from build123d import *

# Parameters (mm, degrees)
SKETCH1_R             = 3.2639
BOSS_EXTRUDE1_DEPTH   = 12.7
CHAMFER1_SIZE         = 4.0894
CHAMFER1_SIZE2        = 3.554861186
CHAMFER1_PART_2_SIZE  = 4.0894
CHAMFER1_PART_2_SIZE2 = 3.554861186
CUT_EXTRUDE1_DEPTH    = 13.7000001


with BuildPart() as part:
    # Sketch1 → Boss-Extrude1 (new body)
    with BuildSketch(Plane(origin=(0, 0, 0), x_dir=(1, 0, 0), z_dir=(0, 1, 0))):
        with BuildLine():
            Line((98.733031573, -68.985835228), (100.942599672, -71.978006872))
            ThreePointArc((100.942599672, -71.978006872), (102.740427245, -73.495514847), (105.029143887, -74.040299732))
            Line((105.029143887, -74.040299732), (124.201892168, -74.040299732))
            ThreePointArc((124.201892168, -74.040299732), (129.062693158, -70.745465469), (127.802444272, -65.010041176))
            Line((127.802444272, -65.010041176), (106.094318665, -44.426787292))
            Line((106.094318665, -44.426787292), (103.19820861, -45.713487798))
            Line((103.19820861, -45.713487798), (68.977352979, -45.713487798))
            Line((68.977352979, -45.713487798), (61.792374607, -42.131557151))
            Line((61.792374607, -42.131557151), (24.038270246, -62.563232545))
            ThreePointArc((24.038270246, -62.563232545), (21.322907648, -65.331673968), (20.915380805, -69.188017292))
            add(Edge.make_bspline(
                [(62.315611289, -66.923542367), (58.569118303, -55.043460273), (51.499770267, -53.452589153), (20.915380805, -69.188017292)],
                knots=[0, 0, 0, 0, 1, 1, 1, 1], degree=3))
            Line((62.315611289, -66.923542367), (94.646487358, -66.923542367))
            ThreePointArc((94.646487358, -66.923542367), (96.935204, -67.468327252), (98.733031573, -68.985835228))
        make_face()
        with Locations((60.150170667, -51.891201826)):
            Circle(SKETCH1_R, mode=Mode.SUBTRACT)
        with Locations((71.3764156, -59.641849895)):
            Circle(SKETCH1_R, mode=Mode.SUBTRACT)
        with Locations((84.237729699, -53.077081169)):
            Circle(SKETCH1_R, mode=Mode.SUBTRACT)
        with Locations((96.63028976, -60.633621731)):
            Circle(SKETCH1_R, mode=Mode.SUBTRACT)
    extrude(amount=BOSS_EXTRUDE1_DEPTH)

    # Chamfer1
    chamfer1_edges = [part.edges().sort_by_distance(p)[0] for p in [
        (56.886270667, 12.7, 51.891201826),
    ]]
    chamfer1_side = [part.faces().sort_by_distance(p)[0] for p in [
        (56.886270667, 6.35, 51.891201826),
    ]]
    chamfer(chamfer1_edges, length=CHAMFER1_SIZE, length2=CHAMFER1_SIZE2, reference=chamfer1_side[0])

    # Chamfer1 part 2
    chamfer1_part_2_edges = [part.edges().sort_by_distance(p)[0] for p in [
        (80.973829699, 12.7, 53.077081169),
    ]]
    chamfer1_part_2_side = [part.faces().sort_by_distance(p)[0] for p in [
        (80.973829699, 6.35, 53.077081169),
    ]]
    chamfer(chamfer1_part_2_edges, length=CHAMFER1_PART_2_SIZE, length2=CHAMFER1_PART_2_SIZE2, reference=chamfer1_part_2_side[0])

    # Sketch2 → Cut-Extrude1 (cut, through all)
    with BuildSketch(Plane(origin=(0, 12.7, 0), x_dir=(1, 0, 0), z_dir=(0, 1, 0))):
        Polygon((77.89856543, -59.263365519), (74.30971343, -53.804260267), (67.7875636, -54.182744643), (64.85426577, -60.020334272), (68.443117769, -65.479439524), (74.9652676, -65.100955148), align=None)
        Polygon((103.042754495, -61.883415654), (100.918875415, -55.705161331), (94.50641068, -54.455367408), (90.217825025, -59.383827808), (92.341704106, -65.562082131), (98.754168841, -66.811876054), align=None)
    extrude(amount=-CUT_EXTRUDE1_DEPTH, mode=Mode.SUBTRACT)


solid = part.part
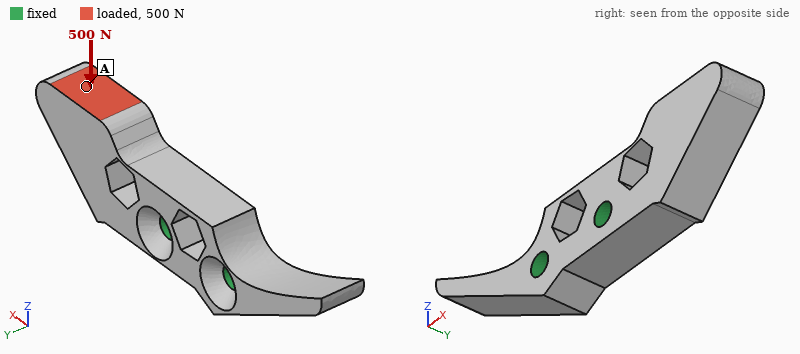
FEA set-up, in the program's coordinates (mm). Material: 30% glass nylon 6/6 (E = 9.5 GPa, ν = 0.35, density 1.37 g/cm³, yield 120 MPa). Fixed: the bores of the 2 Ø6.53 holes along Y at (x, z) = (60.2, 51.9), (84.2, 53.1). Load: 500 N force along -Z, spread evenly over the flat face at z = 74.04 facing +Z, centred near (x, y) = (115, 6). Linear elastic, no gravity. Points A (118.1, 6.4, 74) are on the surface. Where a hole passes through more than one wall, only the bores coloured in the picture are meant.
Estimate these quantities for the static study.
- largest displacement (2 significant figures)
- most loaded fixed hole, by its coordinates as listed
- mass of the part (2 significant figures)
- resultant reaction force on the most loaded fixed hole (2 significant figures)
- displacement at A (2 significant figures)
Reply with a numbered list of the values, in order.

1. 0.29 mm
2. (84.2, 53.1)
3. 25 g
4. 710 N
5. 0.24 mm
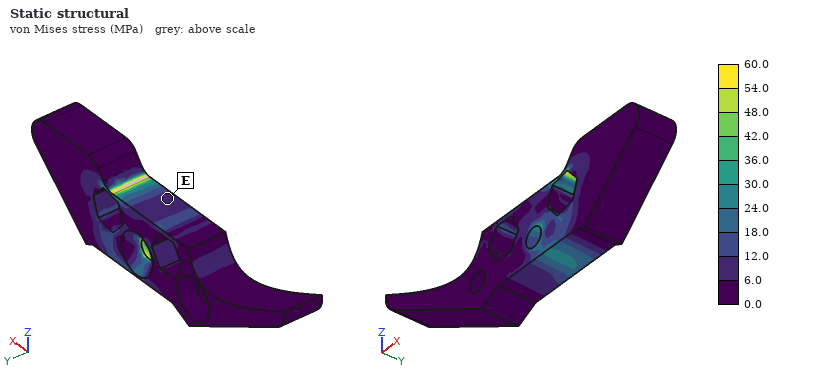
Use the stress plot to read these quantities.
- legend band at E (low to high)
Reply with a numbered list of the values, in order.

1. 6.0 to 12.0 MPa
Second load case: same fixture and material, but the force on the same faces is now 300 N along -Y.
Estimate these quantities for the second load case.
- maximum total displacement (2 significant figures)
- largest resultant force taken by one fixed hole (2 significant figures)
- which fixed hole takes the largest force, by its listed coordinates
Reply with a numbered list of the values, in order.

1. 0.49 mm
2. 410 N
3. (84.2, 53.1)
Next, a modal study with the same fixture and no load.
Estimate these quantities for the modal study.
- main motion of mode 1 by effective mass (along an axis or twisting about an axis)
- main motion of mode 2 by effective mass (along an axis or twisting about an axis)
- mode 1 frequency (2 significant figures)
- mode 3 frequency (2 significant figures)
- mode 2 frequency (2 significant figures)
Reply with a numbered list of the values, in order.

1. along Y
2. along Z
3. 1800 Hz
4. 2800 Hz
5. 2500 Hz
